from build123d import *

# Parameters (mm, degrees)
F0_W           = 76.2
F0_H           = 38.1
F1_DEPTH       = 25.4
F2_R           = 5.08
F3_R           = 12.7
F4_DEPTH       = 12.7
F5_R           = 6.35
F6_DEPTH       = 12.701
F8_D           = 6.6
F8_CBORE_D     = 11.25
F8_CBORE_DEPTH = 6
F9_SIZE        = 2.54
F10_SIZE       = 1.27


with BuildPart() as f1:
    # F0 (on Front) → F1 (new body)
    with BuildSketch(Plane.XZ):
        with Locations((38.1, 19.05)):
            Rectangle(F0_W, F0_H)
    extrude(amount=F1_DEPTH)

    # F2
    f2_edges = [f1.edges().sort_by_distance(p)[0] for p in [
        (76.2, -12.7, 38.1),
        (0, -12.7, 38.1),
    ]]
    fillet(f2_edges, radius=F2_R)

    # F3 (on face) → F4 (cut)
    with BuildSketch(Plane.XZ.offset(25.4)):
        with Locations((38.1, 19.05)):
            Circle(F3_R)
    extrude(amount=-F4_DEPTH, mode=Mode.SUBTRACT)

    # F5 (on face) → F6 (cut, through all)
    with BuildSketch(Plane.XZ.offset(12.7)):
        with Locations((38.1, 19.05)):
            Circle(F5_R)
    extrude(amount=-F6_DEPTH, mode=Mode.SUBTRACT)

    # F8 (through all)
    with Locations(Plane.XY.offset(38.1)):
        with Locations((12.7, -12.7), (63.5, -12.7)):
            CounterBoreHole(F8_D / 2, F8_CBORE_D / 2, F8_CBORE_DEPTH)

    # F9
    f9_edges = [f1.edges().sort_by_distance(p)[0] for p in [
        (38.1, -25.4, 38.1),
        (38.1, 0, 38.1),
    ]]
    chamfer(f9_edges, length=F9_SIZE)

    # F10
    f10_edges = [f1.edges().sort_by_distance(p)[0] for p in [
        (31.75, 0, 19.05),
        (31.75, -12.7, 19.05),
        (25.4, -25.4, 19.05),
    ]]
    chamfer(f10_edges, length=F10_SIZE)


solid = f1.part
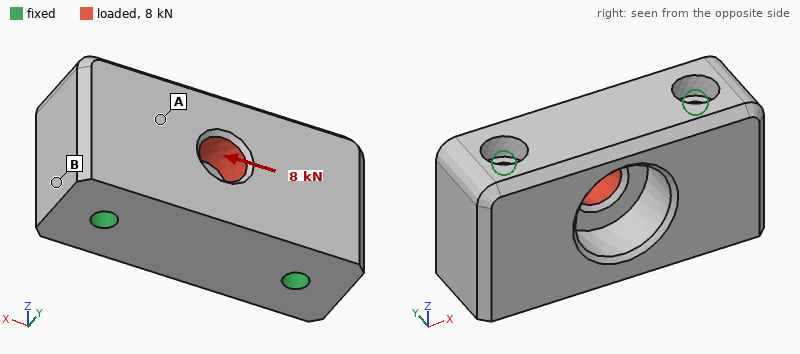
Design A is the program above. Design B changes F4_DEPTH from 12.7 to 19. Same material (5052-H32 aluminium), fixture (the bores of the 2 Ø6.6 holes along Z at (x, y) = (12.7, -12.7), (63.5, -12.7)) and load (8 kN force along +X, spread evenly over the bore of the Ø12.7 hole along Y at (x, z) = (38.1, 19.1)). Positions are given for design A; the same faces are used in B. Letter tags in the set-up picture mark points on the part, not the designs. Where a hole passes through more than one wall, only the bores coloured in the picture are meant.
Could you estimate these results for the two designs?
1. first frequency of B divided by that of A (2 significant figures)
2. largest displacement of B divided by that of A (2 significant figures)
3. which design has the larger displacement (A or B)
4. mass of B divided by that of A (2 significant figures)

1.0
1.9
B
0.96
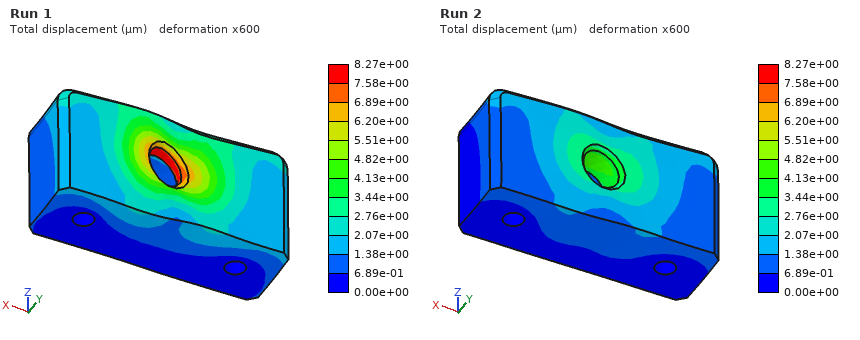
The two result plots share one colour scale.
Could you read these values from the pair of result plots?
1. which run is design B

Run 1
